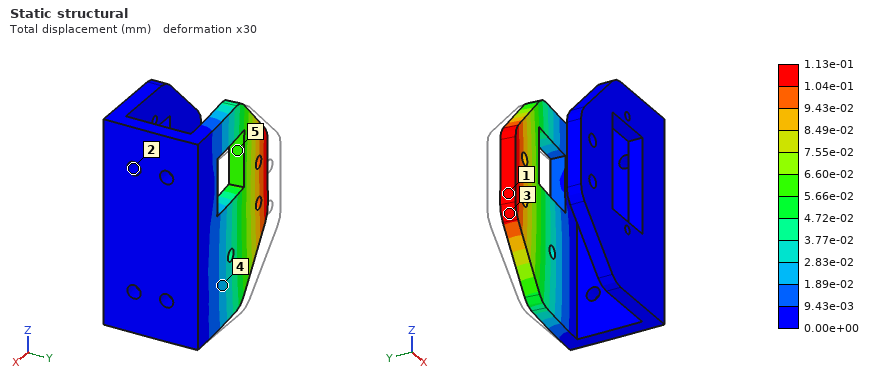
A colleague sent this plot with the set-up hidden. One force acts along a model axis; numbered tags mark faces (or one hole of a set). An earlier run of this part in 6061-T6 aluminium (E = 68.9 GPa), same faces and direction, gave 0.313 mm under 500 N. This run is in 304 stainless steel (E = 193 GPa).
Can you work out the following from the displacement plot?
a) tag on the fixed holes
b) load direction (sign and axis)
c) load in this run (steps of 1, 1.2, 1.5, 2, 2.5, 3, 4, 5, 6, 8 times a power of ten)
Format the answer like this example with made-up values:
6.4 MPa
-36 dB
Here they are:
2
-Y
500 N
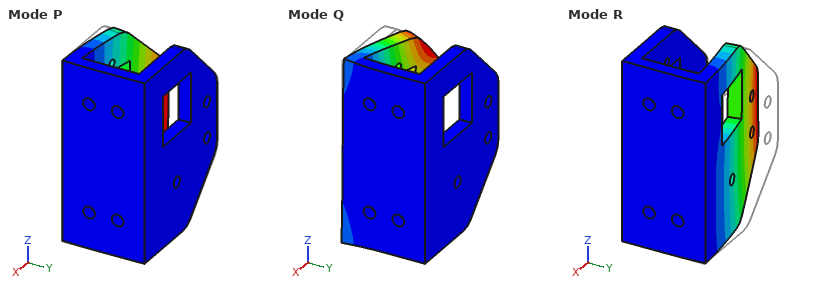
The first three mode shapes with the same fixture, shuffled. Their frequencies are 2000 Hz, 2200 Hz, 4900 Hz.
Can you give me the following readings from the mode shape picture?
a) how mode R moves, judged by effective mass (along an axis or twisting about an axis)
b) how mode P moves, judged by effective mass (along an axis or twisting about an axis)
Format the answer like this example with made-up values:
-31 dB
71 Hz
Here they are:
along Y
along Y
